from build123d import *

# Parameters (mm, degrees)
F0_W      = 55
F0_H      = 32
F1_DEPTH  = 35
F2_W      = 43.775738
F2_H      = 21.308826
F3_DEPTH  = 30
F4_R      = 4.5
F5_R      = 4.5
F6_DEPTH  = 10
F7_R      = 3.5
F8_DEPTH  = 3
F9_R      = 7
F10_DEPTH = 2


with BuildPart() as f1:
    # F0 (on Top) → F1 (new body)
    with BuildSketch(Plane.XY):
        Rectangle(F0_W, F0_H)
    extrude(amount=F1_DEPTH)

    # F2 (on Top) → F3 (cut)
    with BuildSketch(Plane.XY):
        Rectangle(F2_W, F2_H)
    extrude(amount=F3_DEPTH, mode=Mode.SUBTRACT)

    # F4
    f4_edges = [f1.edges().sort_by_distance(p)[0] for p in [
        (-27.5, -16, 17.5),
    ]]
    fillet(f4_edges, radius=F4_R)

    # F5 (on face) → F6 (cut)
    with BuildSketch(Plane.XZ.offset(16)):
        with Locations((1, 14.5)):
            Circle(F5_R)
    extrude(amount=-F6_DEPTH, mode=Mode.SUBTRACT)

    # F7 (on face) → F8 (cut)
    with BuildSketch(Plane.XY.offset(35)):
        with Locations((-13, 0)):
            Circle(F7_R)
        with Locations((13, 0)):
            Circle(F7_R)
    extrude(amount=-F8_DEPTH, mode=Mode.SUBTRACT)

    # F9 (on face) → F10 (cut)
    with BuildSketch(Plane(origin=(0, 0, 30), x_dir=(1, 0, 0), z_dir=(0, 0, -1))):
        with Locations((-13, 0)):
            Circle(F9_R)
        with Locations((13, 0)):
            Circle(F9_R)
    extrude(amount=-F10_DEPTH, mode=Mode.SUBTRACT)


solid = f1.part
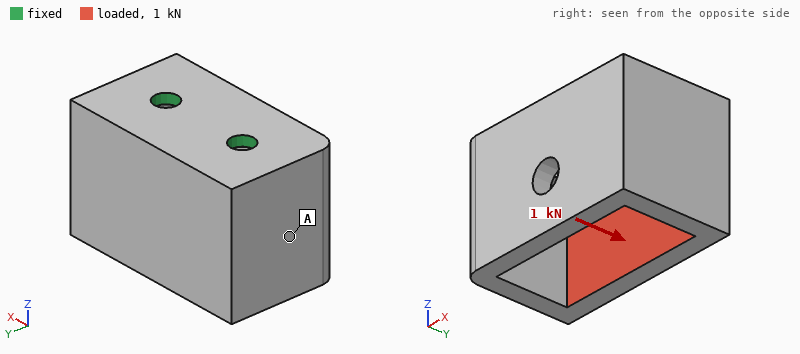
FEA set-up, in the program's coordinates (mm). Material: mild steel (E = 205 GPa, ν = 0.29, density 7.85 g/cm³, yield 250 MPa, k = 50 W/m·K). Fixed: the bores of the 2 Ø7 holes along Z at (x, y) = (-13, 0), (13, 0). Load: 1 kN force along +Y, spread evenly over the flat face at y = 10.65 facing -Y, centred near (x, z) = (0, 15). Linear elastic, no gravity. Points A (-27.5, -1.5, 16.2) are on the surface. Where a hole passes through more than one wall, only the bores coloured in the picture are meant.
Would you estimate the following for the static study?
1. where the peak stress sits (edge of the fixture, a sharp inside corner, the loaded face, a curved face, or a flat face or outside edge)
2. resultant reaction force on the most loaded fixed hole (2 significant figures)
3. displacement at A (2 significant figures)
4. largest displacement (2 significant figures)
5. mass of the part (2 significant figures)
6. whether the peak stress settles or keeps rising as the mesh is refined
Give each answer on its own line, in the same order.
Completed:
edge of the fixture
510 N
16 µm
40 µm
250 g
keeps rising
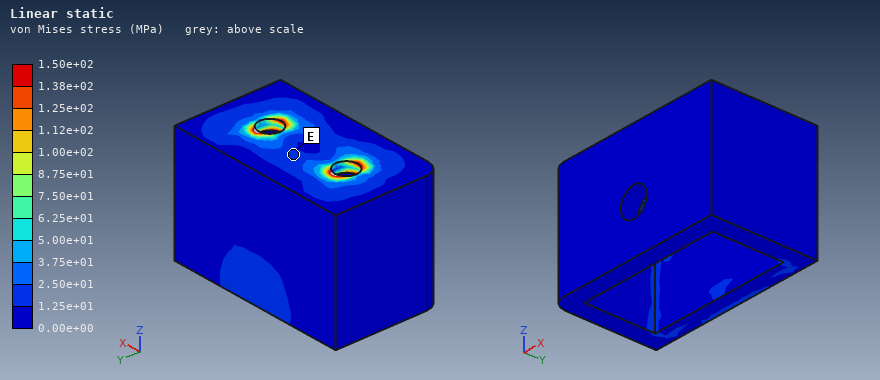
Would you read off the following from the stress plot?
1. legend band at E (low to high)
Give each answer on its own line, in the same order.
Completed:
1.25e+01 to 2.50e+01 MPa
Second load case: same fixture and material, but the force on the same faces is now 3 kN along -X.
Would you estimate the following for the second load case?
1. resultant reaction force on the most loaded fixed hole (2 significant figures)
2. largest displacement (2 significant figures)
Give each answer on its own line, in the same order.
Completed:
2.5 kN
25 µm
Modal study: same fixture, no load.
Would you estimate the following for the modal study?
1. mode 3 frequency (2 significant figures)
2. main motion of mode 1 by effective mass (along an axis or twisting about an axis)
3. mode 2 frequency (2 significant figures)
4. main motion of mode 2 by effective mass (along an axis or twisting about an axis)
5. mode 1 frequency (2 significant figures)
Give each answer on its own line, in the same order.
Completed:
5900 Hz
along Y
4900 Hz
along X
2200 Hz
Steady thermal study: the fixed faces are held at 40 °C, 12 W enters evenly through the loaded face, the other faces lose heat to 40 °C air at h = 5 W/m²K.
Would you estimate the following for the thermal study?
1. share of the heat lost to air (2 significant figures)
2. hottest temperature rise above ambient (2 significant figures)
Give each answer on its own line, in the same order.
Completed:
4.5 %
19 K
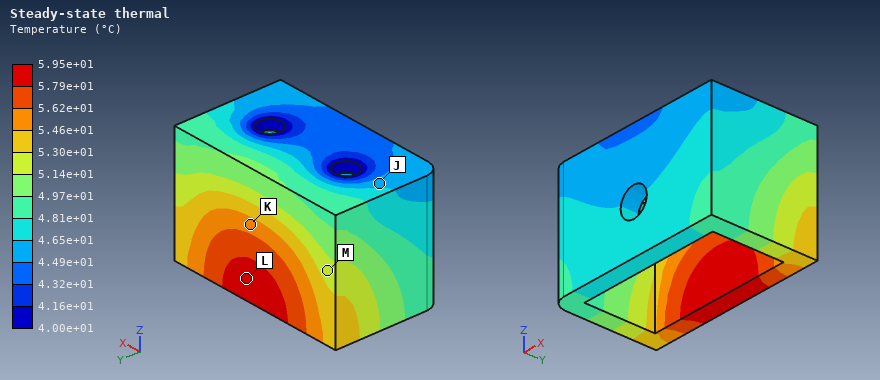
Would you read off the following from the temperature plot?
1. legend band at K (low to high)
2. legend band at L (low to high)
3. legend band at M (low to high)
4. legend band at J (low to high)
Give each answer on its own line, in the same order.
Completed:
5.46e+01 to 5.62e+01 °C
5.79e+01 to 5.95e+01 °C
5.14e+01 to 5.30e+01 °C
4.49e+01 to 4.65e+01 °C
